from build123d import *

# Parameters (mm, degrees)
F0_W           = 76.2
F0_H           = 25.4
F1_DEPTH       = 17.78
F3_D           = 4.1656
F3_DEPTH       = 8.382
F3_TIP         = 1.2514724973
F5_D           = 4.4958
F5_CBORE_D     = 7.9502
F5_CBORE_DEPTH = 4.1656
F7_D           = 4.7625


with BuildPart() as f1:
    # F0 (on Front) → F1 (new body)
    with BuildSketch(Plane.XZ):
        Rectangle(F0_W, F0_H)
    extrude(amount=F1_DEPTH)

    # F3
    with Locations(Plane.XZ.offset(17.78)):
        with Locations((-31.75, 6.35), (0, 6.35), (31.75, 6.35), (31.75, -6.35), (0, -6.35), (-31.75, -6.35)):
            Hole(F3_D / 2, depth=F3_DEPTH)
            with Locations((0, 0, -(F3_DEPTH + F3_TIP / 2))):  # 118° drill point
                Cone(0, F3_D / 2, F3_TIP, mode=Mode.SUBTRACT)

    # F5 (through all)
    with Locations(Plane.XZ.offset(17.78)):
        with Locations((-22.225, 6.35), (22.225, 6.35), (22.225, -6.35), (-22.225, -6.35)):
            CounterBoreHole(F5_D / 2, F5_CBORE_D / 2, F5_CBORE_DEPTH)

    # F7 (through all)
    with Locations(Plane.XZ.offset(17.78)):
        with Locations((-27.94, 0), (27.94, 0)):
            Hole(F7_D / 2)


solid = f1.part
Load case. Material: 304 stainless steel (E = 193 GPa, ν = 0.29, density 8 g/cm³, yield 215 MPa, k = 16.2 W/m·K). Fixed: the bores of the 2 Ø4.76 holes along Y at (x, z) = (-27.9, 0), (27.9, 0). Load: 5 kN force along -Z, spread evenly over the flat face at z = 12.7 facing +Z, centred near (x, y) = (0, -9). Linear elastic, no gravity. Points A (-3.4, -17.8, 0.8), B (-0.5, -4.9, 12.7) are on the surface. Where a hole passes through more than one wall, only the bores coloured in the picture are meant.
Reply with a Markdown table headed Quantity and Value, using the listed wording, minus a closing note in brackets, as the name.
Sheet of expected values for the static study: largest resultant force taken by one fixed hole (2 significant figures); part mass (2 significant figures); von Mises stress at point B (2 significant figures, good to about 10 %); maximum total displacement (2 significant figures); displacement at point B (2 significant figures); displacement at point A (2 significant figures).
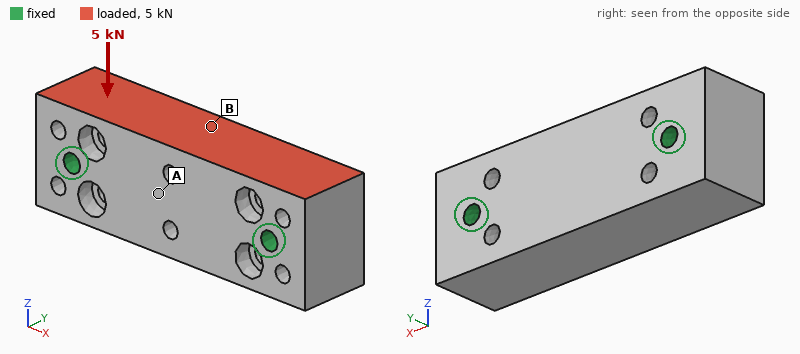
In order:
| Quantity | Value |
|---|---|
| largest resultant force taken by one fixed hole | 2.5 kN |
| part mass | 250 g |
| von Mises stress at point B | 9.2 MPa |
| maximum total displacement | 2.6 µm |
| displacement at point B | 2.3 µm |
| displacement at point A | 2.4 µm |
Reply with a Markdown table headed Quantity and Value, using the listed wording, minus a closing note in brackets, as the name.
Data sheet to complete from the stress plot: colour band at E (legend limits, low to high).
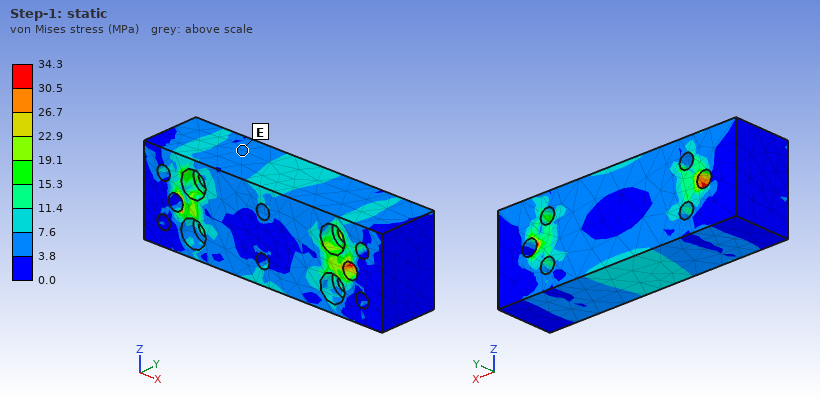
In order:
| Quantity | Value |
|---|---|
| colour band at E | 3.8 to 7.6 MPa |
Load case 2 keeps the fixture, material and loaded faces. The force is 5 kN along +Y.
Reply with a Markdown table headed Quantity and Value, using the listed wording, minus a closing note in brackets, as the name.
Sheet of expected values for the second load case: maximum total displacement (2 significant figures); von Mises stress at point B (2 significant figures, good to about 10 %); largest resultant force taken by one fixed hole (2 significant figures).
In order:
| Quantity | Value |
|---|---|
| maximum total displacement | 7.6 µm |
| von Mises stress at point B | 7.8 MPa |
| largest resultant force taken by one fixed hole | 2.5 kN |
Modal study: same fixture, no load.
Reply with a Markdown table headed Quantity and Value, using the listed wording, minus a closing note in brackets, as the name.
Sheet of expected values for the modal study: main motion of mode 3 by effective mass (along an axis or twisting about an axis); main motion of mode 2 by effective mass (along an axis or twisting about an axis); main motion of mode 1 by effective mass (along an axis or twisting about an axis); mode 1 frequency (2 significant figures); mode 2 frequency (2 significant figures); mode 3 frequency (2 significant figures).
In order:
| Quantity | Value |
|---|---|
| main motion of mode 3 by effective mass | twisting about X |
| main motion of mode 2 by effective mass | along Y |
| main motion of mode 1 by effective mass | along Z |
| mode 1 frequency | 15 kHz |
| mode 2 frequency | 16 kHz |
| mode 3 frequency | 18 kHz |
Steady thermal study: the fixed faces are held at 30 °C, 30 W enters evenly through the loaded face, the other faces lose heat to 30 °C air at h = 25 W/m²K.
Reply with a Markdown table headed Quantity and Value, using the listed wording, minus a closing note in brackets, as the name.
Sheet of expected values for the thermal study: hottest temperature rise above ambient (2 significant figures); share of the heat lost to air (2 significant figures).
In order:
| Quantity | Value |
|---|---|
| hottest temperature rise above ambient | 41 K |
| share of the heat lost to air | 10 % |
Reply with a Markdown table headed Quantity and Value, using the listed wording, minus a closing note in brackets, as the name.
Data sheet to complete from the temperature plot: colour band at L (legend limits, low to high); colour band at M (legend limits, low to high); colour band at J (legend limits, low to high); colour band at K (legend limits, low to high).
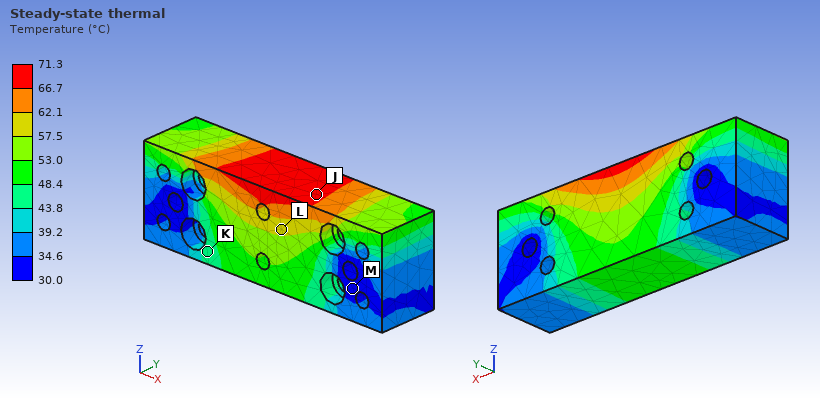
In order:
| Quantity | Value |
|---|---|
| colour band at L | 57.5 to 62.1 °C |
| colour band at M | 30.0 to 34.6 °C |
| colour band at J | 66.7 to 71.3 °C |
| colour band at K | 43.8 to 48.4 °C |
